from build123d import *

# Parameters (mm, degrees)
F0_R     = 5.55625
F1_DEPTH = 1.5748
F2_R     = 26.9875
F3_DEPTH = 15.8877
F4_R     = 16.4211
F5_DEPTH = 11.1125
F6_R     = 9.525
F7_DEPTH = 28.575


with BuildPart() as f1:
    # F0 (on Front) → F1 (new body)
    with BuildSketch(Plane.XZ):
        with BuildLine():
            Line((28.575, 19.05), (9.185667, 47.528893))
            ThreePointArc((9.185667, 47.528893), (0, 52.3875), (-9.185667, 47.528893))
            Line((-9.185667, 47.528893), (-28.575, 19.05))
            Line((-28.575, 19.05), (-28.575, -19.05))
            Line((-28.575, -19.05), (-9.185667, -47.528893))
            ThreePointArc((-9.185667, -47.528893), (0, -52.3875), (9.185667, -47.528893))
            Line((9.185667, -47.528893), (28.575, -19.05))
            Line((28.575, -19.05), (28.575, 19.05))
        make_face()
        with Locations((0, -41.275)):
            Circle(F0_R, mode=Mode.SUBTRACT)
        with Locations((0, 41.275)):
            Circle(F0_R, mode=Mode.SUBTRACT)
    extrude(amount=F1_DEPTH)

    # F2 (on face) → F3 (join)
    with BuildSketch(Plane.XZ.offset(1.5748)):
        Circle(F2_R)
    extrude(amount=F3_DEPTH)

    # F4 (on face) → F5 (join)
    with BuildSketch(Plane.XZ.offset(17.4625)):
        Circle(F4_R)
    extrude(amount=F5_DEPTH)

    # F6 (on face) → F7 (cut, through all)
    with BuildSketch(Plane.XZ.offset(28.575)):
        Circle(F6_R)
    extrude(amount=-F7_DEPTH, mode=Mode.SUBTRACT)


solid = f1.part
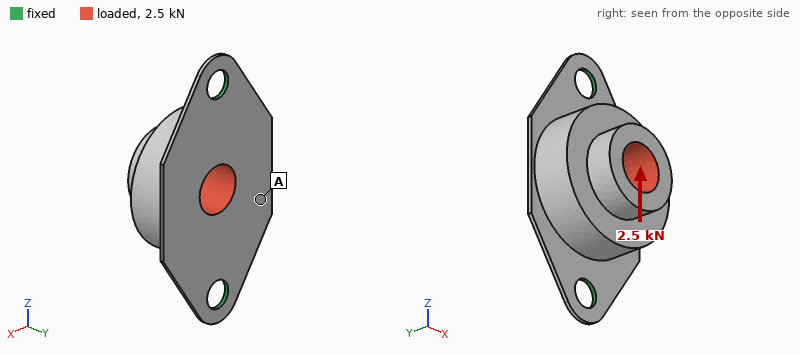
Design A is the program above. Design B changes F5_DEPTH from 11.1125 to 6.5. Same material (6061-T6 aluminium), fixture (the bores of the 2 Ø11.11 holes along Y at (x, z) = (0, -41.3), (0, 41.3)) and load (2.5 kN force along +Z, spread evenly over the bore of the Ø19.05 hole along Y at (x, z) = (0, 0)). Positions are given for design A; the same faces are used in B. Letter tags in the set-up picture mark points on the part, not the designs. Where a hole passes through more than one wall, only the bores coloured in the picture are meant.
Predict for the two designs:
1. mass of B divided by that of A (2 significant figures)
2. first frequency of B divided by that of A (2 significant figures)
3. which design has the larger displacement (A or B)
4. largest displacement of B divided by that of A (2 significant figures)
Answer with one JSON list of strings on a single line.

["0.94", "1.1", "A", "0.78"]
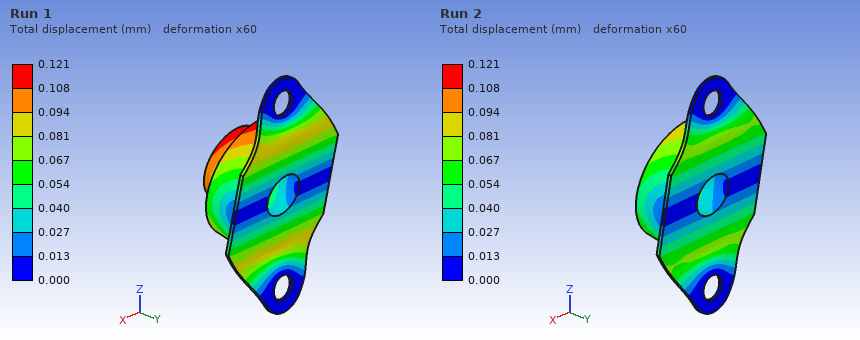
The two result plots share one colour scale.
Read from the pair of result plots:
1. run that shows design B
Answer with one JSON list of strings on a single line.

["Run 2"]
